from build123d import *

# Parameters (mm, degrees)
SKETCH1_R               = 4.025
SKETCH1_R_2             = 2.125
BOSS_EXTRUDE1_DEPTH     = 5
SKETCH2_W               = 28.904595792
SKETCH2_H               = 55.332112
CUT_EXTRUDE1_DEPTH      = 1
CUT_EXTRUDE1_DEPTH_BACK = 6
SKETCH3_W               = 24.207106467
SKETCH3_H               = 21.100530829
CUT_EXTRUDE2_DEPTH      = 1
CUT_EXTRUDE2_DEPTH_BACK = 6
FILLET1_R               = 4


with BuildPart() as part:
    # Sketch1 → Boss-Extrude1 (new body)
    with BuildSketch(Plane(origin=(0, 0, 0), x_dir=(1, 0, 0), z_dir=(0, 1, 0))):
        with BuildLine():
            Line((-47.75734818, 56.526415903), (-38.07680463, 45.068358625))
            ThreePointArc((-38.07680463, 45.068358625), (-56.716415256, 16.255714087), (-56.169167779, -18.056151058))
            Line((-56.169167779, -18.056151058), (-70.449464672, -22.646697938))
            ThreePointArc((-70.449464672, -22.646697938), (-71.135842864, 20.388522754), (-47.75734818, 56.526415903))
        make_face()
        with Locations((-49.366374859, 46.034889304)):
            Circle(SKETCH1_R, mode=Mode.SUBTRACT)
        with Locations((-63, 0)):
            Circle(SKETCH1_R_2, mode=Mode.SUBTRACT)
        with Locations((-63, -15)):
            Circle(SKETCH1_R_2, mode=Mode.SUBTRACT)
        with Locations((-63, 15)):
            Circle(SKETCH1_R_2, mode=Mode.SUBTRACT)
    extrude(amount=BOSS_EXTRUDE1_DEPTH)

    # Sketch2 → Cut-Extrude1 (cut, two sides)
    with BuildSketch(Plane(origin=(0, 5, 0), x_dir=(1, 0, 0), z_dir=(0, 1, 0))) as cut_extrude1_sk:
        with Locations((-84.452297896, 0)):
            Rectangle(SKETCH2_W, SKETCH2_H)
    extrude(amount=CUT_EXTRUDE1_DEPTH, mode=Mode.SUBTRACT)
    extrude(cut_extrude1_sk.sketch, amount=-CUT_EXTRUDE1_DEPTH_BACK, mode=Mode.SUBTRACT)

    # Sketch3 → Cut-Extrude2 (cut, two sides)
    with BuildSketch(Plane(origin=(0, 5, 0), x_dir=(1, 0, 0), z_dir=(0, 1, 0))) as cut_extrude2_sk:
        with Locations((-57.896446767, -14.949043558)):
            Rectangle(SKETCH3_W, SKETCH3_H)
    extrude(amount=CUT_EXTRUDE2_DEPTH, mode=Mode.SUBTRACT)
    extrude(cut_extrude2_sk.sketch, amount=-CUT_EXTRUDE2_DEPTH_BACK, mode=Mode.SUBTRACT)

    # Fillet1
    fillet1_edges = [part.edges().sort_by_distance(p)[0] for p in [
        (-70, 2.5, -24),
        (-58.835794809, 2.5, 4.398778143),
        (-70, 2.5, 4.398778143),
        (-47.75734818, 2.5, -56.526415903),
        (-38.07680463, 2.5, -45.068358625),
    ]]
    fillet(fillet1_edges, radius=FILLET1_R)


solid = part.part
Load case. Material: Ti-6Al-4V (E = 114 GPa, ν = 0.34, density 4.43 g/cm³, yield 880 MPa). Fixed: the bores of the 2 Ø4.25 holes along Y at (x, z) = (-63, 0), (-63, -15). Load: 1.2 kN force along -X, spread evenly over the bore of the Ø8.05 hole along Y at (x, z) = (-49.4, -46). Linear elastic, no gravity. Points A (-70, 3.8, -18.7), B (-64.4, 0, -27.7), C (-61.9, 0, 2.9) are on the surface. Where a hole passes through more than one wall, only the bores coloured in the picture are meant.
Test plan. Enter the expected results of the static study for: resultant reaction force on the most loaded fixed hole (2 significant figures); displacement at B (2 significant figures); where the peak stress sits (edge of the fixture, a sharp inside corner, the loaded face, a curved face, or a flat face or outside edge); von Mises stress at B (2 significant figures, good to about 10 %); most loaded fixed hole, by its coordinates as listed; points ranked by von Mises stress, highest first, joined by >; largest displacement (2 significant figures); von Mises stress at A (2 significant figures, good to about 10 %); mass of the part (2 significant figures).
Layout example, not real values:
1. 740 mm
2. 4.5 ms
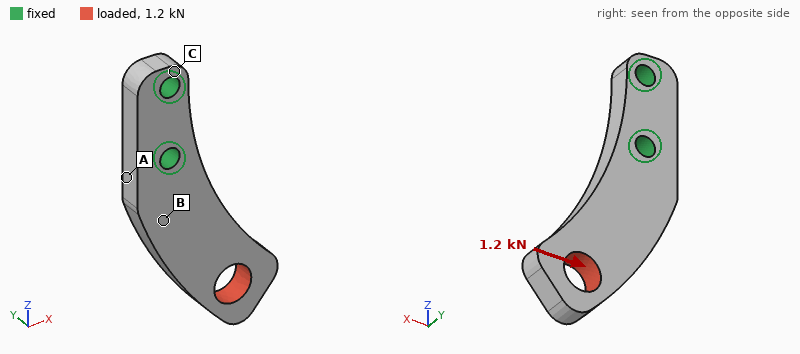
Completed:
1. 2.3 kN
2. 0.044 mm
3. edge of the fixture
4. 77 MPa
5. (-63, -15)
6. A > B > C
7. 0.22 mm
8. 200 MPa
9. 17 g
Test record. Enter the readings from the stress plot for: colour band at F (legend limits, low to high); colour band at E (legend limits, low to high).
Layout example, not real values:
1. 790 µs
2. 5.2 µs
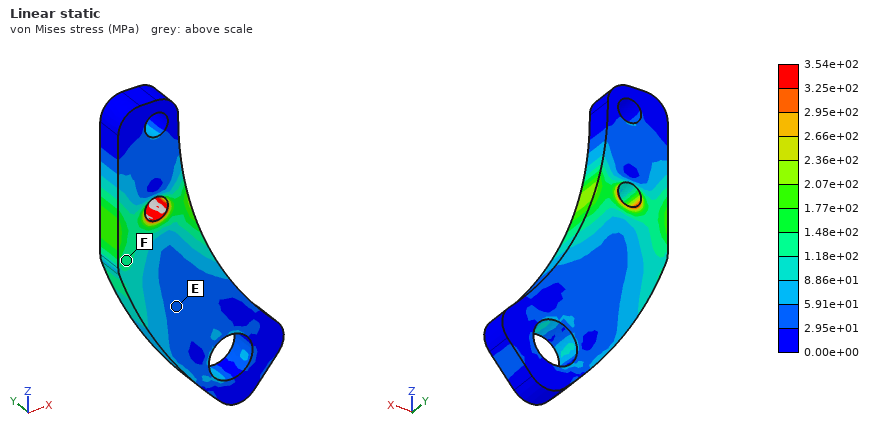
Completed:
1. 1.18e+02 to 1.48e+02 MPa
2. 2.95e+01 to 5.91e+01 MPa
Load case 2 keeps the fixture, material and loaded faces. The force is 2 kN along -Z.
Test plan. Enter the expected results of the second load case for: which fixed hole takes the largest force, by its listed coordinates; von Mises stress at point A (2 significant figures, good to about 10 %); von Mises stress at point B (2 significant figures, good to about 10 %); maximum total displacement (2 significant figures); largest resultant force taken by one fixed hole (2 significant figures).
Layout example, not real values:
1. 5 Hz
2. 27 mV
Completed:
1. (-63, -15)
2. 140 MPa
3. 44 MPa
4. 0.19 mm
5. 2.3 kN
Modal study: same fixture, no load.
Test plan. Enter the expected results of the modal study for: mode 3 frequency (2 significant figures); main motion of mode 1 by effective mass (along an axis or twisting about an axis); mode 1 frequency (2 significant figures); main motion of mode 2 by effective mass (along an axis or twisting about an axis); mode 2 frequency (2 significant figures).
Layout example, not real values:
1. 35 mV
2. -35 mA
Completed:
1. 10 kHz
2. along Y
3. 2700 Hz
4. along X
5. 5500 Hz
